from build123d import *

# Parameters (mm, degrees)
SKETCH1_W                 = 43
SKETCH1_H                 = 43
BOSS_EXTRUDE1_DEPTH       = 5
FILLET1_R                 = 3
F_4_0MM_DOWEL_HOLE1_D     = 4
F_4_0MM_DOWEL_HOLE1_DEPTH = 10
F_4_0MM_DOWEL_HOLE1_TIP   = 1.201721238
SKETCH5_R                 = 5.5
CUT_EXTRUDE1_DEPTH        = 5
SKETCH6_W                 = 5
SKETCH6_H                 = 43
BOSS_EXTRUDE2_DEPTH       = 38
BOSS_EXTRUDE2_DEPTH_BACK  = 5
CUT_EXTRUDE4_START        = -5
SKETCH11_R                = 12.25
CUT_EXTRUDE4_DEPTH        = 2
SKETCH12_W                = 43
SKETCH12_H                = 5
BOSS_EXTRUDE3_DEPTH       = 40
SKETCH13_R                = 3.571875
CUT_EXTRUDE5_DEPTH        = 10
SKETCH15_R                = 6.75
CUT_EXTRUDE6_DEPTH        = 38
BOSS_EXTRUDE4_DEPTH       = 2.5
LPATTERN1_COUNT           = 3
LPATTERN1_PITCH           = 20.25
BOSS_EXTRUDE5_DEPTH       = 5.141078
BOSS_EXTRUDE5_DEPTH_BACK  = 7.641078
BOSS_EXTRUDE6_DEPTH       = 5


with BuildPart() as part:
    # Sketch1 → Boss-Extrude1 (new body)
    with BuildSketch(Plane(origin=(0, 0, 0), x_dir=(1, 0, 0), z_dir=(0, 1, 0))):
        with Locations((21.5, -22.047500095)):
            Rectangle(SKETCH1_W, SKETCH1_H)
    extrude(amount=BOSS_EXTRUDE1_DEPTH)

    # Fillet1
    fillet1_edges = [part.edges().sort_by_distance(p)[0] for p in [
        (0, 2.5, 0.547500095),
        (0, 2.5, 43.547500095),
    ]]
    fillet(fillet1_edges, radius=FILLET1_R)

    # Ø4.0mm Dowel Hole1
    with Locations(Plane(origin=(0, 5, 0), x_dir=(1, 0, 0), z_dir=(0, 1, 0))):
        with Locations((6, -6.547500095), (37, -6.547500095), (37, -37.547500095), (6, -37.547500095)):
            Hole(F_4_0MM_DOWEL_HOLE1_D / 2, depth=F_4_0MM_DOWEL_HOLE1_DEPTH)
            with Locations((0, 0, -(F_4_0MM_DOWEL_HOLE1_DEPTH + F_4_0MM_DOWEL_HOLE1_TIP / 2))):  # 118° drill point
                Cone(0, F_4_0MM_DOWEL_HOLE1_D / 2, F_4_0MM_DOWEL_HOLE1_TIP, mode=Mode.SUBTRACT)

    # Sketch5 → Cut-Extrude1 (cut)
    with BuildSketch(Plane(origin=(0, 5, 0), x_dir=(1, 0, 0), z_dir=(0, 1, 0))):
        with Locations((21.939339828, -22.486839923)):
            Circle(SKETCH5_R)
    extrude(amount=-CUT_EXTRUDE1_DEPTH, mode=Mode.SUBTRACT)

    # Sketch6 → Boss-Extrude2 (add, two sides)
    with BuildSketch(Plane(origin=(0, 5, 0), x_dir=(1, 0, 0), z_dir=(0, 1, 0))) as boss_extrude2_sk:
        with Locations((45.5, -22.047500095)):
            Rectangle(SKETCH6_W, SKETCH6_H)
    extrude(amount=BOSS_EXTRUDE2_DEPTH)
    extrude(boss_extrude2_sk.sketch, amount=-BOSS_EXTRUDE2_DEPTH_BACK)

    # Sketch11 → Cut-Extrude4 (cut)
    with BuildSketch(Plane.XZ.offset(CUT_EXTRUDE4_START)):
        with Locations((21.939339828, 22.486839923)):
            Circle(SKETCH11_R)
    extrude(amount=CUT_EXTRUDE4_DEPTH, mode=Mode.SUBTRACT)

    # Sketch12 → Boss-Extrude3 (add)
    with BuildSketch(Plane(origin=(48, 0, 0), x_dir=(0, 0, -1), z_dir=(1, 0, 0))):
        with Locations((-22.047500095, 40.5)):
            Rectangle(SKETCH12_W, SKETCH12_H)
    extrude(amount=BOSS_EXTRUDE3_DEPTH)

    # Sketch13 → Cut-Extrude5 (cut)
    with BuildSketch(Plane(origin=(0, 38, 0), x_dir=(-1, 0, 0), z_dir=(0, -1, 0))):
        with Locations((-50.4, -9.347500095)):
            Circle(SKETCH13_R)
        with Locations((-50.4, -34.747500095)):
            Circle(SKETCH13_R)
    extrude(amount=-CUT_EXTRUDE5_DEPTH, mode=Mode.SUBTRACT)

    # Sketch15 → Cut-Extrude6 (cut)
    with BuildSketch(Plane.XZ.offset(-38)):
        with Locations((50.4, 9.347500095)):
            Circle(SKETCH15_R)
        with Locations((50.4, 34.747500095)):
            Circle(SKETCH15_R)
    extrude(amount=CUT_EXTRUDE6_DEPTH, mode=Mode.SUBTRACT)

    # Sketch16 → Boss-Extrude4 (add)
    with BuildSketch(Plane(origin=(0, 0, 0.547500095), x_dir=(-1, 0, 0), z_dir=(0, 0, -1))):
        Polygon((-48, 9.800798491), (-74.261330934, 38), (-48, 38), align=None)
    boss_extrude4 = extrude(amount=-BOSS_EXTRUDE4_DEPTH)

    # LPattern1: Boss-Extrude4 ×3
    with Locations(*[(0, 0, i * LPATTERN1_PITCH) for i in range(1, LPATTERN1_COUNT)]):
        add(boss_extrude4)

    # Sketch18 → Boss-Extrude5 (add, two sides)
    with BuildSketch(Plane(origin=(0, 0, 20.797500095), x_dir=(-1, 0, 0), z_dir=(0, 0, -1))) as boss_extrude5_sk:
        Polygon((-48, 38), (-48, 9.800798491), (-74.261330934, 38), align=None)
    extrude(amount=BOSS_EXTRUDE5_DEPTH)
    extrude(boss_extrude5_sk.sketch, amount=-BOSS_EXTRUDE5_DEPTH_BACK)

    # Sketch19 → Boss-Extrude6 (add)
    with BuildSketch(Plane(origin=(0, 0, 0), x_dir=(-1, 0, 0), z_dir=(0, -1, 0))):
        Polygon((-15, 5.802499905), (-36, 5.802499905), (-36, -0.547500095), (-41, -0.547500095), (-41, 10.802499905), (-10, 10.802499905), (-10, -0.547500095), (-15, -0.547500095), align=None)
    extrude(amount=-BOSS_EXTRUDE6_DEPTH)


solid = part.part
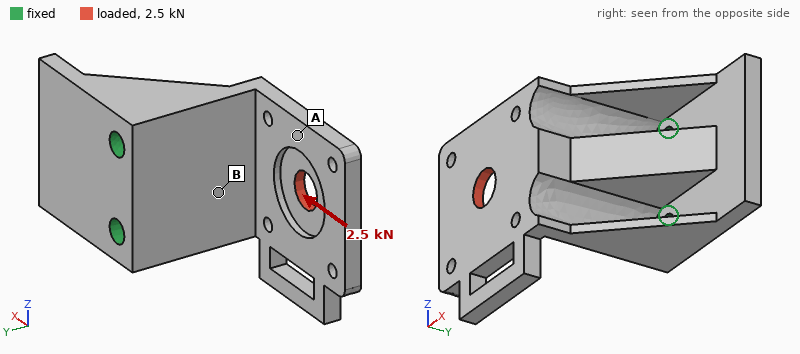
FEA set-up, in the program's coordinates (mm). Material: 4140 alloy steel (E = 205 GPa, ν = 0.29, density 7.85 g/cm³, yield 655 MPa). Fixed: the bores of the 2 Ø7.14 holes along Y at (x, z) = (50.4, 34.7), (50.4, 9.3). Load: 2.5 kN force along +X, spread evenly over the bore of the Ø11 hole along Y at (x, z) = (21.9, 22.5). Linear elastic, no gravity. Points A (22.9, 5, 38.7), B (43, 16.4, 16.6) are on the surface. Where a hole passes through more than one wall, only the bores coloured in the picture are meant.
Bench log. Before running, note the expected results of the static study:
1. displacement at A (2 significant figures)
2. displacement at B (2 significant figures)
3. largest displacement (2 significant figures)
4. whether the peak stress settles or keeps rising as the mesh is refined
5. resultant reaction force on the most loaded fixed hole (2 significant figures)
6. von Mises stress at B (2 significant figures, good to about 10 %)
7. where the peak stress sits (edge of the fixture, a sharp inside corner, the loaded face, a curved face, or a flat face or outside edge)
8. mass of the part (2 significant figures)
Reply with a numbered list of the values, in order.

1. 0.17 mm
2. 0.048 mm
3. 0.30 mm
4. keeps rising
5. 1.3 kN
6. 83 MPa
7. a sharp inside corner
8. 230 g
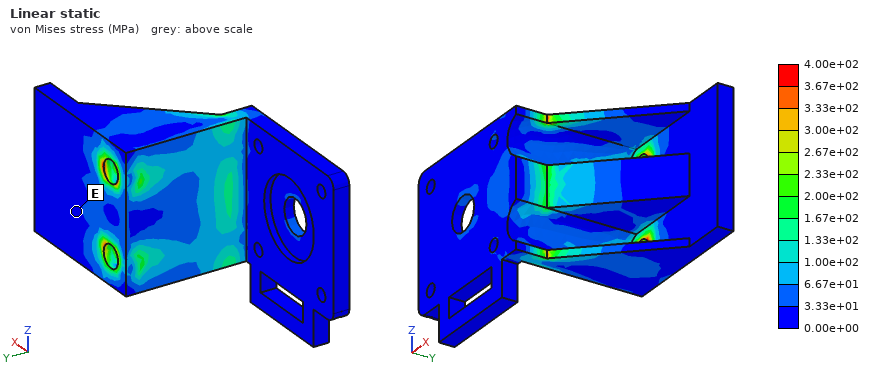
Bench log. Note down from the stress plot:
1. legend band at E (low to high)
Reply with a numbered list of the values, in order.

1. 0.00e+00 to 3.33e+01 MPa
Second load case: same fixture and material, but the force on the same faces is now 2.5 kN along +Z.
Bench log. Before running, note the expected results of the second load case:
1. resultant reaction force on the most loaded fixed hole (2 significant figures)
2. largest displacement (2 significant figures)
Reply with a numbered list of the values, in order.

1. 3.9 kN
2. 0.21 mm
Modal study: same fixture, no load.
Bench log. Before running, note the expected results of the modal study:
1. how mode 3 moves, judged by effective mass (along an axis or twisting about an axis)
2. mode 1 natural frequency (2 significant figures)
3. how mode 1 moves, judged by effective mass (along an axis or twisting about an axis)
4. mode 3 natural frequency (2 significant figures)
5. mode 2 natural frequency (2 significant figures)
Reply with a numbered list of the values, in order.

1. along X
2. 1100 Hz
3. along Y
4. 3000 Hz
5. 2200 Hz
